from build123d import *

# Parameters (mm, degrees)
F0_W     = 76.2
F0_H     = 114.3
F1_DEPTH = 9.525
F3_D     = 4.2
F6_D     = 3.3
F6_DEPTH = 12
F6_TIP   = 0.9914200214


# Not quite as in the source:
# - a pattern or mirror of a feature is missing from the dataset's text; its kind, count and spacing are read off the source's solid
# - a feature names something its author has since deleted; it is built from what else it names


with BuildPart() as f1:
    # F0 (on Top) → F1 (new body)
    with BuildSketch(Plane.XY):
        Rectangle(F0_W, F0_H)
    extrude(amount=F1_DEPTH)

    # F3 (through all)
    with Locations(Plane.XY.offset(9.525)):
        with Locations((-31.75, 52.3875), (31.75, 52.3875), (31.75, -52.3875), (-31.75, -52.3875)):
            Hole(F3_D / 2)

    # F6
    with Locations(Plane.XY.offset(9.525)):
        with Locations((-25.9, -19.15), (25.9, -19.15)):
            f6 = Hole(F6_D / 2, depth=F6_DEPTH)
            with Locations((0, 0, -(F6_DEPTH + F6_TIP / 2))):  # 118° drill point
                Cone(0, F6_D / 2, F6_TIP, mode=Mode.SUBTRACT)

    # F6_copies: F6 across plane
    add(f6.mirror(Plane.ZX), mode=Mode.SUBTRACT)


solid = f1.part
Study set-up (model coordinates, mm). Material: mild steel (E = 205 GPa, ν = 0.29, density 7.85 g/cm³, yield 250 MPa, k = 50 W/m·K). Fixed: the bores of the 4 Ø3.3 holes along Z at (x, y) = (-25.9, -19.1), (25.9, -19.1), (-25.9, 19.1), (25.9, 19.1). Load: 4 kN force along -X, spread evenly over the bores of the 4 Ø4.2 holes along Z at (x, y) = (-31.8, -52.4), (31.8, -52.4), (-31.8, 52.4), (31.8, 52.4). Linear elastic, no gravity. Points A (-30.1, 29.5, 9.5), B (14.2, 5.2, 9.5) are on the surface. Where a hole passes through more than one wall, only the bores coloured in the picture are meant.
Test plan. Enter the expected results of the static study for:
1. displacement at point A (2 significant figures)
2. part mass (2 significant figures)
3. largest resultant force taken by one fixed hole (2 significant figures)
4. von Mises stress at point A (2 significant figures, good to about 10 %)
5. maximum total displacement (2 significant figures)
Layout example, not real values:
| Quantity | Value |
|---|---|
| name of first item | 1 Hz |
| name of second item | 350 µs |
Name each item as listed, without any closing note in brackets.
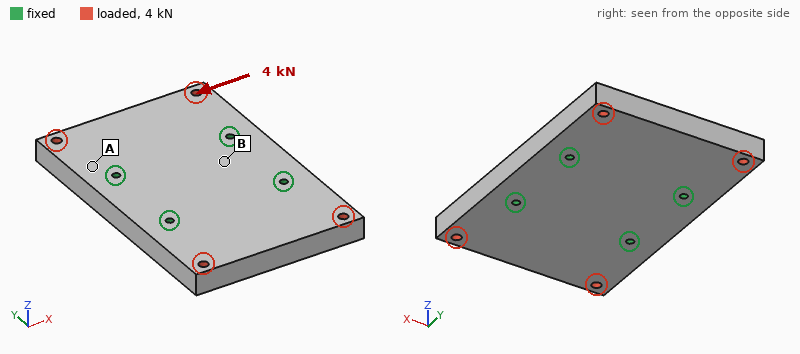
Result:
| Quantity | Value |
|---|---|
| displacement at point A | 0.84 µm |
| part mass | 640 g |
| largest resultant force taken by one fixed hole | 1.2 kN |
| von Mises stress at point A | 4.3 MPa |
| maximum total displacement | 3.2 µm |
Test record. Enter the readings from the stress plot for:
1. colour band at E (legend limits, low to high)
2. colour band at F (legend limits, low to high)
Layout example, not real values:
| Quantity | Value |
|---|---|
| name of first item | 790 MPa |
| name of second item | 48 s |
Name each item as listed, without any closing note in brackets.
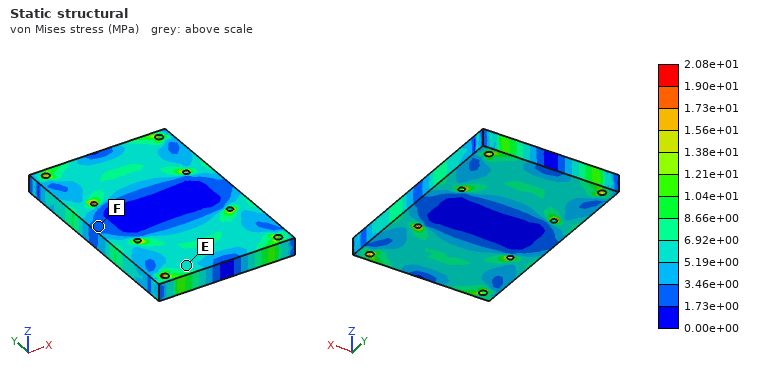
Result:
| Quantity | Value |
|---|---|
| colour band at E | 5.19e+00 to 6.92e+00 MPa |
| colour band at F | 1.73e+00 to 3.46e+00 MPa |
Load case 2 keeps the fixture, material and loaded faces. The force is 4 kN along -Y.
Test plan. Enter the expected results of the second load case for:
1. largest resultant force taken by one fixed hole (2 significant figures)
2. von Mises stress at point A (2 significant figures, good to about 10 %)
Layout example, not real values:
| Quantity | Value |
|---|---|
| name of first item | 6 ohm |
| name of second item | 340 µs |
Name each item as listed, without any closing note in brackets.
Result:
| Quantity | Value |
|---|---|
| largest resultant force taken by one fixed hole | 1.0 kN |
| von Mises stress at point A | 6.0 MPa |
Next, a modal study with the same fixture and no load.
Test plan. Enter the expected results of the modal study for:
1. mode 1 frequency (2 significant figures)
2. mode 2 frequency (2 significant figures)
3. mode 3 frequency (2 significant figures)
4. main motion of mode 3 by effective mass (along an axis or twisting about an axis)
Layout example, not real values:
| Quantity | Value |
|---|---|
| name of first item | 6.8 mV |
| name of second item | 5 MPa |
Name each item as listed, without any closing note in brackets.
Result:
| Quantity | Value |
|---|---|
| mode 1 frequency | 4200 Hz |
| mode 2 frequency | 4300 Hz |
| mode 3 frequency | 7200 Hz |
| main motion of mode 3 by effective mass | twisting about Y |
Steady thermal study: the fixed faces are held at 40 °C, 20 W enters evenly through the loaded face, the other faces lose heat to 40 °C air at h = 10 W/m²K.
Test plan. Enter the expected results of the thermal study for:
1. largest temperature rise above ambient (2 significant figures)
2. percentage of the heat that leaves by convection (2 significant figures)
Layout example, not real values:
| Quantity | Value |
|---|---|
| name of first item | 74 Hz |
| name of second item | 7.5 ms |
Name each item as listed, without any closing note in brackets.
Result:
| Quantity | Value |
|---|---|
| largest temperature rise above ambient | 17 K |
| percentage of the heat that leaves by convection | 6.2 % |
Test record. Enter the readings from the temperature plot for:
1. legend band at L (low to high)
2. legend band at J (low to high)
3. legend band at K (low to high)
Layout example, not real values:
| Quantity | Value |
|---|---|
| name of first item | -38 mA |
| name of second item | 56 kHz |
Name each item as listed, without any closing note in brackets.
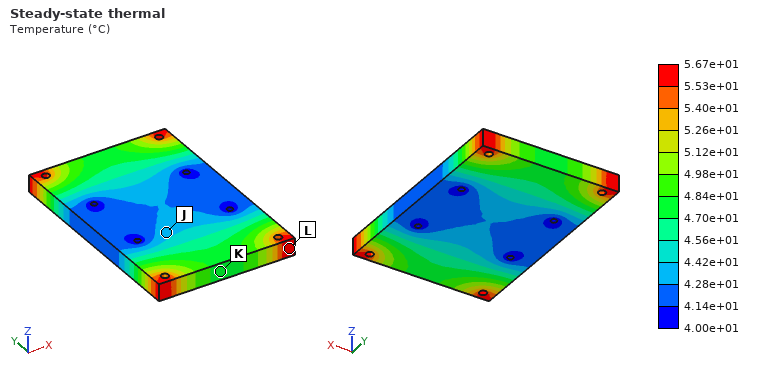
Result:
| Quantity | Value |
|---|---|
| legend band at L | 5.53e+01 to 5.67e+01 °C |
| legend band at J | 4.28e+01 to 4.42e+01 °C |
| legend band at K | 4.70e+01 to 4.84e+01 °C |
